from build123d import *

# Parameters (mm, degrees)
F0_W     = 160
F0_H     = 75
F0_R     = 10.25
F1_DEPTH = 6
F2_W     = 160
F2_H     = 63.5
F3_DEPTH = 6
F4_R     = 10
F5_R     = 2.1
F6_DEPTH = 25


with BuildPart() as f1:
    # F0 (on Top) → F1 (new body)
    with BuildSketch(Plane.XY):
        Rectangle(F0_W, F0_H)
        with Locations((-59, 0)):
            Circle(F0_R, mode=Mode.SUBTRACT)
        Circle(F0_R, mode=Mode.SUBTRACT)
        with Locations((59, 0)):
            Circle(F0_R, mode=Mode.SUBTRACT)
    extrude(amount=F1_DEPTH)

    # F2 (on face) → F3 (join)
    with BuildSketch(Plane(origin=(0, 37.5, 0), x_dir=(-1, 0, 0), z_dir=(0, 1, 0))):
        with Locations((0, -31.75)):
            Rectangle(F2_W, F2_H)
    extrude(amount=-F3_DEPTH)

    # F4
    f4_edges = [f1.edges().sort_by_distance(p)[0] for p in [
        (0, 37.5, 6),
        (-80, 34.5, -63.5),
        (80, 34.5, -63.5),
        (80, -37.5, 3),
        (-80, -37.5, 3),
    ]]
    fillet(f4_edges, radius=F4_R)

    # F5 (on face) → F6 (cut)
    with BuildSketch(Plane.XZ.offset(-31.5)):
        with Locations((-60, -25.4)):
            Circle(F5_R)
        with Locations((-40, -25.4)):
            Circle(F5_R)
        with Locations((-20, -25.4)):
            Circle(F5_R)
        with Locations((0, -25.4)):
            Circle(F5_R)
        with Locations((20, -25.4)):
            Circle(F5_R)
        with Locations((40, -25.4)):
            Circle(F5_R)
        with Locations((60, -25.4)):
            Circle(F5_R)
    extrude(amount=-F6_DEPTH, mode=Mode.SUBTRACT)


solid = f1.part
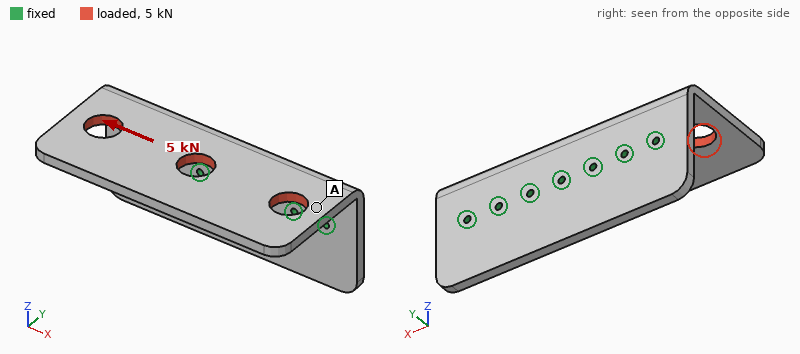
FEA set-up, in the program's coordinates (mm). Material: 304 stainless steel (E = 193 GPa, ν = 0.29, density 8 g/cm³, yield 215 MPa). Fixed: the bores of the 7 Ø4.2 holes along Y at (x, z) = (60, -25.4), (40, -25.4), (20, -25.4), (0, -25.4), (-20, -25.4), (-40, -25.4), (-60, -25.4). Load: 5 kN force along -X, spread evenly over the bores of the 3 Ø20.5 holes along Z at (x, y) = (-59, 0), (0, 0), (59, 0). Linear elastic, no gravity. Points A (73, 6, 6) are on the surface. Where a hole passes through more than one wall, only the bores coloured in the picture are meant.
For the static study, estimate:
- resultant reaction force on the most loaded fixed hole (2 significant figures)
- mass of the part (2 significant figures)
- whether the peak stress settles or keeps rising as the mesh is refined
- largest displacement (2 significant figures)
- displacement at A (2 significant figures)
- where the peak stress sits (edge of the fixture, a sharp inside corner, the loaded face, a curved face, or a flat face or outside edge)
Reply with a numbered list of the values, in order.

1. 1.6 kN
2. 980 g
3. keeps rising
4. 0.13 mm
5. 0.089 mm
6. edge of the fixture
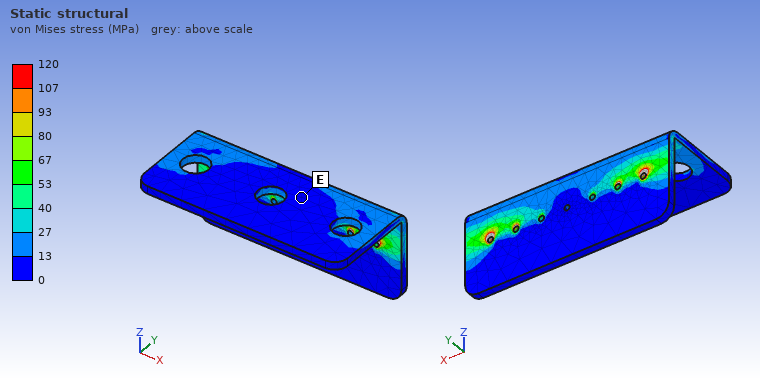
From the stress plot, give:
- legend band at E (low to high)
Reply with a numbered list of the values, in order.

1. 0 to 13 MPa
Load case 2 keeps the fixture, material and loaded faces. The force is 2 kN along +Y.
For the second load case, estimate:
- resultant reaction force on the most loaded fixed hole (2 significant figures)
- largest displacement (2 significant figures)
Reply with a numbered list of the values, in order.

1. 320 N
2. 0.12 mm
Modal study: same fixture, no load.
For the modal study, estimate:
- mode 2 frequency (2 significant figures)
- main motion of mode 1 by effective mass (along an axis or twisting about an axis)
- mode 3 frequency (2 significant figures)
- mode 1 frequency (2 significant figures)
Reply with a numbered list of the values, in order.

1. 960 Hz
2. along Z
3. 1800 Hz
4. 550 Hz
